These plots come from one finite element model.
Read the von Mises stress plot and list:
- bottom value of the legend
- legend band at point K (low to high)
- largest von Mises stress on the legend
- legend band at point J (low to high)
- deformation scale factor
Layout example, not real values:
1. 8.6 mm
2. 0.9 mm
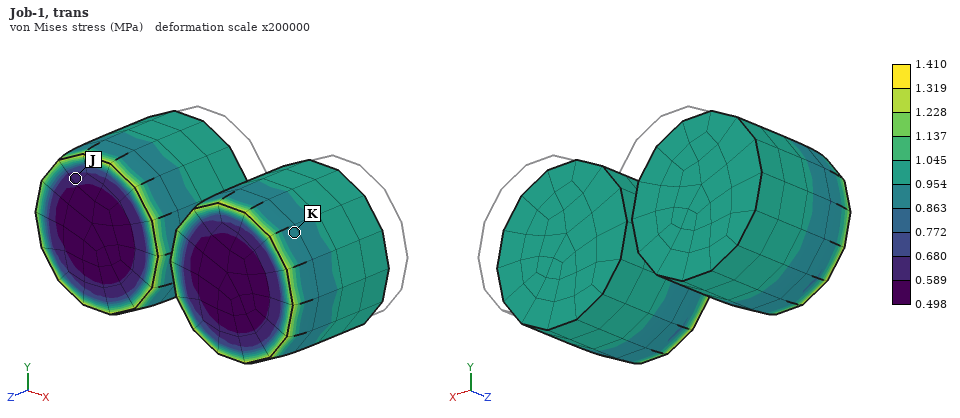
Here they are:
1. 0.498 MPa
2. 0.863 to 0.954 MPa
3. 1.410 MPa
4. 0.589 to 0.680 MPa
5. 200000
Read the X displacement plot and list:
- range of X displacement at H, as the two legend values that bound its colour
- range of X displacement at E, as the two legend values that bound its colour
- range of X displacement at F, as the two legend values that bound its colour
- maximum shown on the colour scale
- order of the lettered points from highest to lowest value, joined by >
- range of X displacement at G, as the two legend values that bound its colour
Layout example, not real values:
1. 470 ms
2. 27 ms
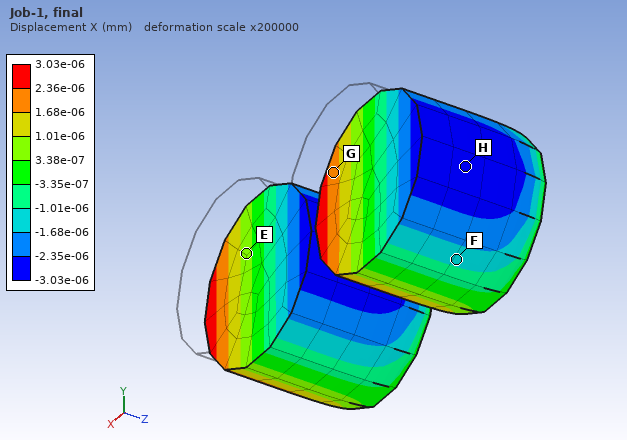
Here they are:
1. -3.03e-06 to -2.35e-06 mm
2. 3.38e-07 to 1.01e-06 mm
3. -1.68e-06 to -1.01e-06 mm
4. 3.03e-06 mm
5. G > E > F > H
6. 1.68e-06 to 2.36e-06 mm
